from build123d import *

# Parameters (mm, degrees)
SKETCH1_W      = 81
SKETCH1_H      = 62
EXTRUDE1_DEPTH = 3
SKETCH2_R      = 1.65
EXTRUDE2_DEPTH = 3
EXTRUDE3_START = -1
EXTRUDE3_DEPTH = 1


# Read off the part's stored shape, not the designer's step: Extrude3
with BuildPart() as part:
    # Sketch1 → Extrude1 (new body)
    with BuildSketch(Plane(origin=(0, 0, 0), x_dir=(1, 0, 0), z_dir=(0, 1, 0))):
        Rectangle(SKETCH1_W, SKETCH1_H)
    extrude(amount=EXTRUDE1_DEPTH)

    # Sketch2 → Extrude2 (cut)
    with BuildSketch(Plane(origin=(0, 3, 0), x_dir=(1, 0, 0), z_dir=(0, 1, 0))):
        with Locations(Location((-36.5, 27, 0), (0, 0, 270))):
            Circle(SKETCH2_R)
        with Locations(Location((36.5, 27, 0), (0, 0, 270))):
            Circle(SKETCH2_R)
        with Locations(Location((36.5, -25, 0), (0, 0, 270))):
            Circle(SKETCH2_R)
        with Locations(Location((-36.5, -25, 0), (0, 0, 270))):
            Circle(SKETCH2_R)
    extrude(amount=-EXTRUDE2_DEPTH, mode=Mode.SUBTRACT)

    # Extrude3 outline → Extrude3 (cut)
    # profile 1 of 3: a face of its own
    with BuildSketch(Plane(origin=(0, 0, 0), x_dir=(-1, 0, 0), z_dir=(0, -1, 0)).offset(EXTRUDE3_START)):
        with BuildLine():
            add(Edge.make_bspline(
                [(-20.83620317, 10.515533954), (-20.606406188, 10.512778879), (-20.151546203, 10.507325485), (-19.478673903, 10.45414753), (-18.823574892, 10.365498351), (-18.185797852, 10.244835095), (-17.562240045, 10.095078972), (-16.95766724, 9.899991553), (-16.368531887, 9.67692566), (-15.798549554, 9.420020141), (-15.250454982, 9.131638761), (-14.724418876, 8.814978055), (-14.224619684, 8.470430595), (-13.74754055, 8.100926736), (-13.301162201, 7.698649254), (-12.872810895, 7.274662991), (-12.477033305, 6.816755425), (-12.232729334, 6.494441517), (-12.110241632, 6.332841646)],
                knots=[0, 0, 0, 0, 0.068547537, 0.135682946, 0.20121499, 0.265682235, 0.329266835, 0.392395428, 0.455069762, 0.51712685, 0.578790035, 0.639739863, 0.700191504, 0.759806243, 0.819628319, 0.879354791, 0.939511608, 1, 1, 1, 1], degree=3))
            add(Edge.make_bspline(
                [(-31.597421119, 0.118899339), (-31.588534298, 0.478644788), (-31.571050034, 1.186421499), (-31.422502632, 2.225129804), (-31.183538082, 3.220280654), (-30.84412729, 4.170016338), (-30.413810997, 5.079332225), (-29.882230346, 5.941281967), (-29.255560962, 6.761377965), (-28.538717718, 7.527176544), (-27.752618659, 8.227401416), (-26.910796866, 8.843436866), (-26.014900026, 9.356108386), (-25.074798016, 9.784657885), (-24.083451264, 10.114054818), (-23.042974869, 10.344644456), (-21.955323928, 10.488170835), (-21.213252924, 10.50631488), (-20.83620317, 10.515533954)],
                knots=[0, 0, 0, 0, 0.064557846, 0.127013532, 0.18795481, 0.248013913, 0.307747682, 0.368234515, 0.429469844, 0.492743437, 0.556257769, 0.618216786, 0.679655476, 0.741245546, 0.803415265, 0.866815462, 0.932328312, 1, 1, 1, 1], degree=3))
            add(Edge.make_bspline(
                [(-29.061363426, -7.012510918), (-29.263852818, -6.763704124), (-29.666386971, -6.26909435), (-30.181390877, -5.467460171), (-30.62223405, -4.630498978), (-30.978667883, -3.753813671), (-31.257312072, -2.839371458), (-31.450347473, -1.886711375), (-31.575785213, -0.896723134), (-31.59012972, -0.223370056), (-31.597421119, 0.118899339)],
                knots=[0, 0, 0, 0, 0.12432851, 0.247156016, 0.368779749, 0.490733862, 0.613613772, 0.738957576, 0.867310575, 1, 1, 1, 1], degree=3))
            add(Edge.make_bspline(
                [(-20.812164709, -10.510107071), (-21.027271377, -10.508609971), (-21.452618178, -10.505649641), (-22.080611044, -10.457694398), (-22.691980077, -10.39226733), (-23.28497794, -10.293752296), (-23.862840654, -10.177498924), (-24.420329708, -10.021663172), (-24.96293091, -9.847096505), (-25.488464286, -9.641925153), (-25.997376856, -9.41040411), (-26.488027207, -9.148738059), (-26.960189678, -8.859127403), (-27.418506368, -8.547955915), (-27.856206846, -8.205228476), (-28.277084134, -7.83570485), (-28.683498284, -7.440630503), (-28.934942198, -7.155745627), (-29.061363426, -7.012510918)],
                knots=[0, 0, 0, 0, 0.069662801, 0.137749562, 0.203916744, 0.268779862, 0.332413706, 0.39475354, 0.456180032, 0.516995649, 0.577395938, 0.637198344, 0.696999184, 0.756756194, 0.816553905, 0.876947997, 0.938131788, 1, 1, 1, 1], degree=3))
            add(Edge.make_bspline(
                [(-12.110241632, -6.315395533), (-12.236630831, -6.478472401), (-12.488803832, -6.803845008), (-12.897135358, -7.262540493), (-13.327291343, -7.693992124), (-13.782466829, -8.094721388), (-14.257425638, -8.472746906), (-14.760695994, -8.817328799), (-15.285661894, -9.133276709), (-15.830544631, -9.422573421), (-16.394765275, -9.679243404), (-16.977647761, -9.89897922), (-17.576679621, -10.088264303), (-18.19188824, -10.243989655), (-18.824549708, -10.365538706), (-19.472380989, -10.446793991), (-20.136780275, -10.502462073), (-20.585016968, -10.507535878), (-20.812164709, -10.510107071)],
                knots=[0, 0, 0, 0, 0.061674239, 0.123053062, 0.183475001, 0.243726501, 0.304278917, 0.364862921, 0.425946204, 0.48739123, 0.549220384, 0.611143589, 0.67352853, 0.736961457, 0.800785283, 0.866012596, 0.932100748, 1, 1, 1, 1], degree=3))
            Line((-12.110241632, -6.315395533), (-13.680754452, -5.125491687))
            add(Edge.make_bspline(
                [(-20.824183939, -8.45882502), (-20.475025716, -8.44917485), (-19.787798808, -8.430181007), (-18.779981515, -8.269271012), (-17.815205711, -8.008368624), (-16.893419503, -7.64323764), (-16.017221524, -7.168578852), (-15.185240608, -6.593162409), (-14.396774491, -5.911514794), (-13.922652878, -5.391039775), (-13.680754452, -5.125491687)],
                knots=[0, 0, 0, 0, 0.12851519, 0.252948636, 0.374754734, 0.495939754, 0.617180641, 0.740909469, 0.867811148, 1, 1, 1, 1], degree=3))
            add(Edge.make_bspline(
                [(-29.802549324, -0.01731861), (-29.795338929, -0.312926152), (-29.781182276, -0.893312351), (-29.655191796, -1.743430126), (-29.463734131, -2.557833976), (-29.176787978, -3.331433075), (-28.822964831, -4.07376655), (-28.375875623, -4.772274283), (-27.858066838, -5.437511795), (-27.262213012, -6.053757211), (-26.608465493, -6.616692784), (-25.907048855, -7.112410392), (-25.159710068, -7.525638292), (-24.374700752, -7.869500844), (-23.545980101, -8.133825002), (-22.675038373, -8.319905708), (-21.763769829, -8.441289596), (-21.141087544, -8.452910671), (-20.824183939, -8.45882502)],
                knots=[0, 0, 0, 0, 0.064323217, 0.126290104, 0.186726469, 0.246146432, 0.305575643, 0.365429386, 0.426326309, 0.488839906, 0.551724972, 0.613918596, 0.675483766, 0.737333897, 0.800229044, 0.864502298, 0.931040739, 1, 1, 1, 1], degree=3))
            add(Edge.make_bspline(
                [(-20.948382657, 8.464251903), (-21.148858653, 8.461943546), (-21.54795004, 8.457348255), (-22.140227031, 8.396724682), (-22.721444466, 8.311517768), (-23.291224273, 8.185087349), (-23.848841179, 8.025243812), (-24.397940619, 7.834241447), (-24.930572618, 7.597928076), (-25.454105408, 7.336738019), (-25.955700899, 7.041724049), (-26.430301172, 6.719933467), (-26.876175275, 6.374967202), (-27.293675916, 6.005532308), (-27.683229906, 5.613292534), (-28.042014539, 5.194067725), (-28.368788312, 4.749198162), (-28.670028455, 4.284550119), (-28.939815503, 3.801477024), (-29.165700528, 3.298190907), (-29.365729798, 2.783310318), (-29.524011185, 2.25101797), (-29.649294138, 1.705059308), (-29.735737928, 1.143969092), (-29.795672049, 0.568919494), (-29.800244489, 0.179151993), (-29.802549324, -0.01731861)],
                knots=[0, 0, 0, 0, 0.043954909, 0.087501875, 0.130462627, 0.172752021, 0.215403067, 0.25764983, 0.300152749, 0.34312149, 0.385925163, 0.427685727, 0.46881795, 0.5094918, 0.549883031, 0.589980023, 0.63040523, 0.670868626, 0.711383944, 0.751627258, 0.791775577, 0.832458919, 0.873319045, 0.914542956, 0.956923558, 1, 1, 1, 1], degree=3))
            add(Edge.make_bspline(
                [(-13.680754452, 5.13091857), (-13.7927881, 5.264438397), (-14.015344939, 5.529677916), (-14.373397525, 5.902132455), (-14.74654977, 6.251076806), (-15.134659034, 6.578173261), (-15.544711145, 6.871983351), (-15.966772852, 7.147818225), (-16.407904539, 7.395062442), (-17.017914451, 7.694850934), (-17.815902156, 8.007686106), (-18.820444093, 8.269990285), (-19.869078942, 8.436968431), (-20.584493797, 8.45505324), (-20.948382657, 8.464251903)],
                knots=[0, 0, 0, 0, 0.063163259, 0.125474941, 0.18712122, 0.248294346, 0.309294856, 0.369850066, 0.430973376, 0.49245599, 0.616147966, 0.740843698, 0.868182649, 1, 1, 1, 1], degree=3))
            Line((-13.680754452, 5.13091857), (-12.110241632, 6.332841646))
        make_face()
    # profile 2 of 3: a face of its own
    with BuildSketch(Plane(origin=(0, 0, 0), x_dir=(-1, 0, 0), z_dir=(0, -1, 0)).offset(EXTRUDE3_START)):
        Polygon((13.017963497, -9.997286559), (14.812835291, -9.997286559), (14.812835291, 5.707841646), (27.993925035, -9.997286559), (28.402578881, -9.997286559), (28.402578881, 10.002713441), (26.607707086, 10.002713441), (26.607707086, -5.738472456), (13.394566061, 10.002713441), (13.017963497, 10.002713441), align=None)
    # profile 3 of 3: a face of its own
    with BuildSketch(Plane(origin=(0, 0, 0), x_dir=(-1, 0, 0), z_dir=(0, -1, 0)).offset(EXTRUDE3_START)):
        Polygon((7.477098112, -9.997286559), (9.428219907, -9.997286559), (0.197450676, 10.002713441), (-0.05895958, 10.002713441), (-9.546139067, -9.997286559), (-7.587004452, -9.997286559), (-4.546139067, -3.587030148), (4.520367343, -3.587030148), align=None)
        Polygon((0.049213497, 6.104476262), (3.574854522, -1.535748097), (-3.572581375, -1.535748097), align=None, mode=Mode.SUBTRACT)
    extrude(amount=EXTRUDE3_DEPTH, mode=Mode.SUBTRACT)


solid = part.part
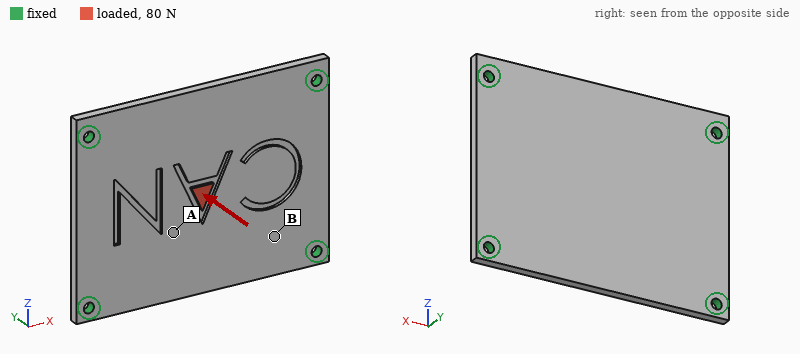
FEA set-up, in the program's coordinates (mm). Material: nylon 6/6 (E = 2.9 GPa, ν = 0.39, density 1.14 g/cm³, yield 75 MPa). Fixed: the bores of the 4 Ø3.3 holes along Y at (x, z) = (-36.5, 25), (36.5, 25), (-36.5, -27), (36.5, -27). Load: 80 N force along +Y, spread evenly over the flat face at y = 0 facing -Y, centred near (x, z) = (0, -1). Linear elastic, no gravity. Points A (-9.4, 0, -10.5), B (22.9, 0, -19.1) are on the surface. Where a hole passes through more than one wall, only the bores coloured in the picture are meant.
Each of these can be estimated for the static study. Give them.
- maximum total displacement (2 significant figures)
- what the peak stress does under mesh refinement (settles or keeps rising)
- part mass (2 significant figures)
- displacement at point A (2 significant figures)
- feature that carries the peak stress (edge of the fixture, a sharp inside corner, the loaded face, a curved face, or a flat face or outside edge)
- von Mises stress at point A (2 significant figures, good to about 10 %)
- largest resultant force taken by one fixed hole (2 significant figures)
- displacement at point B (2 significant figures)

0.85 mm
keeps rising
17 g
0.64 mm
a sharp inside corner
6.3 MPa
24 N
0.26 mm
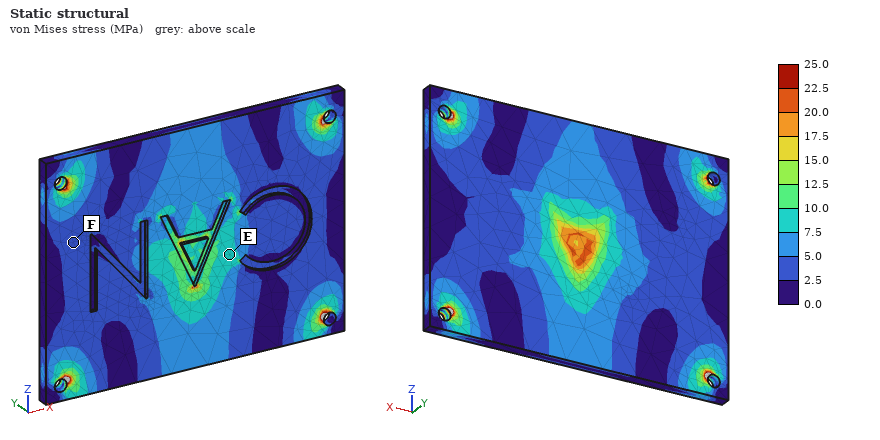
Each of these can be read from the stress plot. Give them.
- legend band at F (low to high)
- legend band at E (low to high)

2.5 to 5.0 MPa
7.5 to 10.0 MPa
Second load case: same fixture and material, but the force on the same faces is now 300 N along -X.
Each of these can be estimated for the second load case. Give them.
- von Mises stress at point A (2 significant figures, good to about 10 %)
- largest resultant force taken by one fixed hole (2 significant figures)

3.7 MPa
85 N
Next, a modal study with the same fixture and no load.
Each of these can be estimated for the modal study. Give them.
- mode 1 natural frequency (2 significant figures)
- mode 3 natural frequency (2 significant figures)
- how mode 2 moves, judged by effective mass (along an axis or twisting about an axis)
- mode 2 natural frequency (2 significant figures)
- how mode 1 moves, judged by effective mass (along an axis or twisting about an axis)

730 Hz
1700 Hz
twisting about X
1100 Hz
along Y
